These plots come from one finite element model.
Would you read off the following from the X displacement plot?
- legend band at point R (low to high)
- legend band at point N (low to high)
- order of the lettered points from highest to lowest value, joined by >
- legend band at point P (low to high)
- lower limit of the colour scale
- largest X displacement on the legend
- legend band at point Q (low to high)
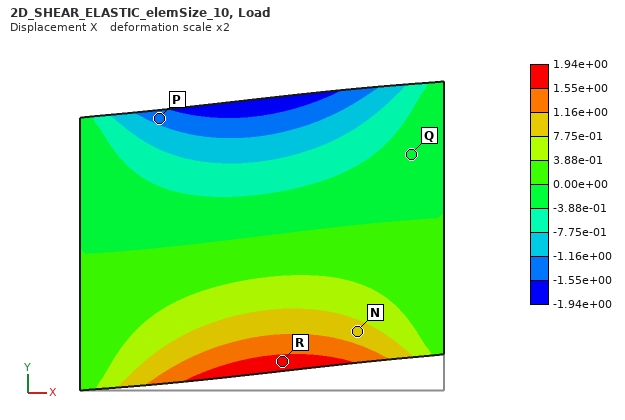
1.55e+00 to 1.94e+00
7.75e-01 to 1.16e+00
R > N > Q > P
-1.55e+00 to -1.16e+00
-1.94e+00
1.94e+00
-3.88e-01 to 0.00e+00
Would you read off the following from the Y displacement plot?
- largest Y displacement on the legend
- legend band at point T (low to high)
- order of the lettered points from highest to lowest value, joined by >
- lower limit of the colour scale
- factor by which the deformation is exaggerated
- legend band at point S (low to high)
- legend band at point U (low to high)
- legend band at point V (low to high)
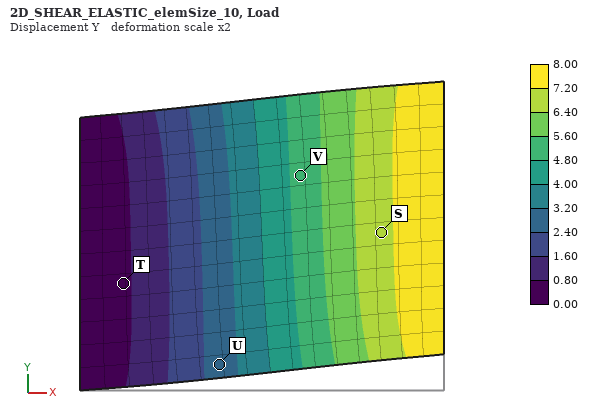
8.00
0.00 to 0.80
S > V > U > T
0.00
2
6.40 to 7.20
2.40 to 3.20
4.80 to 5.60
